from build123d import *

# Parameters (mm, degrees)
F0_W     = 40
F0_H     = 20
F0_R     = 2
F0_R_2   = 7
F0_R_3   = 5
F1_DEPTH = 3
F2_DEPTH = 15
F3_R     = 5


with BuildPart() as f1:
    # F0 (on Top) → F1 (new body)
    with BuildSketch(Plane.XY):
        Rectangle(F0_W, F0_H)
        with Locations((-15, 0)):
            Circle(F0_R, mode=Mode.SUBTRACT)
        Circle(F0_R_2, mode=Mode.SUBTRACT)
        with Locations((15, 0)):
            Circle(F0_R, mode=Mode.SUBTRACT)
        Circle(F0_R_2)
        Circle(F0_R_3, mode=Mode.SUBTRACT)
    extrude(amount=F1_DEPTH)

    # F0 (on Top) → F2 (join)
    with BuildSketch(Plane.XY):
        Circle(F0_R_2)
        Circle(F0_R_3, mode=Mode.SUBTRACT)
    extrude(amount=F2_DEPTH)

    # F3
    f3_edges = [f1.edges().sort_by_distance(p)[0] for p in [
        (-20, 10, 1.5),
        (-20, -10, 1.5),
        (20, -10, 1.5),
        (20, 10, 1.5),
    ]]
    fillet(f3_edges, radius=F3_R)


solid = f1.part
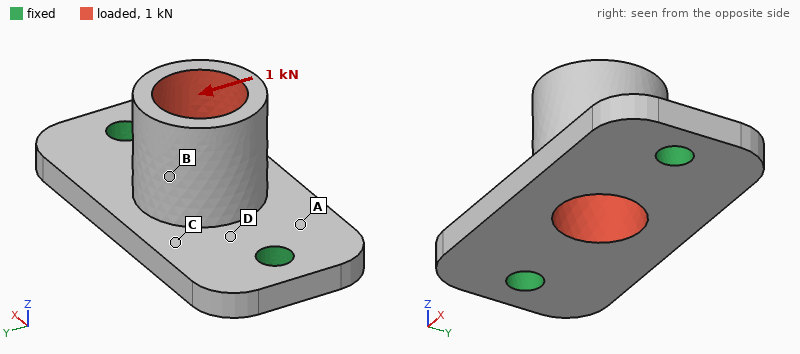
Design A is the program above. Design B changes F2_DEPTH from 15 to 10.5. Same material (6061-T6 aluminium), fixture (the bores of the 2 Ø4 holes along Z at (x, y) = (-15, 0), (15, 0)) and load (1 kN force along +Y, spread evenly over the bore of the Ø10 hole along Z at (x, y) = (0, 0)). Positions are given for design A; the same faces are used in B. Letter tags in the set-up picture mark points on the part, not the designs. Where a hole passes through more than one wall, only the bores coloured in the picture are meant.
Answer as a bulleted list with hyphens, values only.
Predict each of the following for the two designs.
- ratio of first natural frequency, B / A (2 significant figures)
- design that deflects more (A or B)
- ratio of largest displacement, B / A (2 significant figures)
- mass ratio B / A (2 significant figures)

- 1.4
- A
- 0.49
- 0.88
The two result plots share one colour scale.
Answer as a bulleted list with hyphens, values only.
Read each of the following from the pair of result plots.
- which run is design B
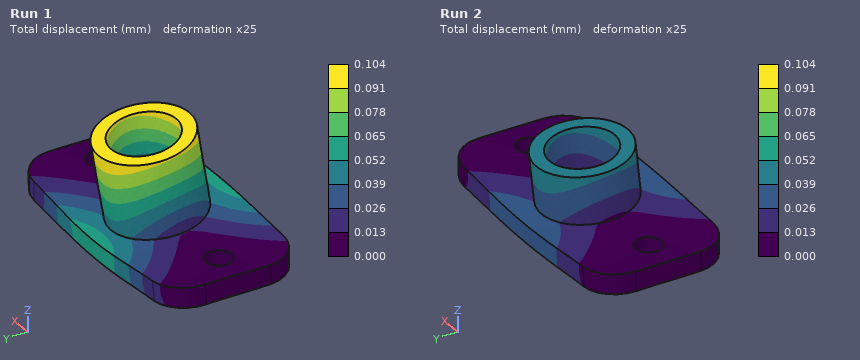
- Run 2
